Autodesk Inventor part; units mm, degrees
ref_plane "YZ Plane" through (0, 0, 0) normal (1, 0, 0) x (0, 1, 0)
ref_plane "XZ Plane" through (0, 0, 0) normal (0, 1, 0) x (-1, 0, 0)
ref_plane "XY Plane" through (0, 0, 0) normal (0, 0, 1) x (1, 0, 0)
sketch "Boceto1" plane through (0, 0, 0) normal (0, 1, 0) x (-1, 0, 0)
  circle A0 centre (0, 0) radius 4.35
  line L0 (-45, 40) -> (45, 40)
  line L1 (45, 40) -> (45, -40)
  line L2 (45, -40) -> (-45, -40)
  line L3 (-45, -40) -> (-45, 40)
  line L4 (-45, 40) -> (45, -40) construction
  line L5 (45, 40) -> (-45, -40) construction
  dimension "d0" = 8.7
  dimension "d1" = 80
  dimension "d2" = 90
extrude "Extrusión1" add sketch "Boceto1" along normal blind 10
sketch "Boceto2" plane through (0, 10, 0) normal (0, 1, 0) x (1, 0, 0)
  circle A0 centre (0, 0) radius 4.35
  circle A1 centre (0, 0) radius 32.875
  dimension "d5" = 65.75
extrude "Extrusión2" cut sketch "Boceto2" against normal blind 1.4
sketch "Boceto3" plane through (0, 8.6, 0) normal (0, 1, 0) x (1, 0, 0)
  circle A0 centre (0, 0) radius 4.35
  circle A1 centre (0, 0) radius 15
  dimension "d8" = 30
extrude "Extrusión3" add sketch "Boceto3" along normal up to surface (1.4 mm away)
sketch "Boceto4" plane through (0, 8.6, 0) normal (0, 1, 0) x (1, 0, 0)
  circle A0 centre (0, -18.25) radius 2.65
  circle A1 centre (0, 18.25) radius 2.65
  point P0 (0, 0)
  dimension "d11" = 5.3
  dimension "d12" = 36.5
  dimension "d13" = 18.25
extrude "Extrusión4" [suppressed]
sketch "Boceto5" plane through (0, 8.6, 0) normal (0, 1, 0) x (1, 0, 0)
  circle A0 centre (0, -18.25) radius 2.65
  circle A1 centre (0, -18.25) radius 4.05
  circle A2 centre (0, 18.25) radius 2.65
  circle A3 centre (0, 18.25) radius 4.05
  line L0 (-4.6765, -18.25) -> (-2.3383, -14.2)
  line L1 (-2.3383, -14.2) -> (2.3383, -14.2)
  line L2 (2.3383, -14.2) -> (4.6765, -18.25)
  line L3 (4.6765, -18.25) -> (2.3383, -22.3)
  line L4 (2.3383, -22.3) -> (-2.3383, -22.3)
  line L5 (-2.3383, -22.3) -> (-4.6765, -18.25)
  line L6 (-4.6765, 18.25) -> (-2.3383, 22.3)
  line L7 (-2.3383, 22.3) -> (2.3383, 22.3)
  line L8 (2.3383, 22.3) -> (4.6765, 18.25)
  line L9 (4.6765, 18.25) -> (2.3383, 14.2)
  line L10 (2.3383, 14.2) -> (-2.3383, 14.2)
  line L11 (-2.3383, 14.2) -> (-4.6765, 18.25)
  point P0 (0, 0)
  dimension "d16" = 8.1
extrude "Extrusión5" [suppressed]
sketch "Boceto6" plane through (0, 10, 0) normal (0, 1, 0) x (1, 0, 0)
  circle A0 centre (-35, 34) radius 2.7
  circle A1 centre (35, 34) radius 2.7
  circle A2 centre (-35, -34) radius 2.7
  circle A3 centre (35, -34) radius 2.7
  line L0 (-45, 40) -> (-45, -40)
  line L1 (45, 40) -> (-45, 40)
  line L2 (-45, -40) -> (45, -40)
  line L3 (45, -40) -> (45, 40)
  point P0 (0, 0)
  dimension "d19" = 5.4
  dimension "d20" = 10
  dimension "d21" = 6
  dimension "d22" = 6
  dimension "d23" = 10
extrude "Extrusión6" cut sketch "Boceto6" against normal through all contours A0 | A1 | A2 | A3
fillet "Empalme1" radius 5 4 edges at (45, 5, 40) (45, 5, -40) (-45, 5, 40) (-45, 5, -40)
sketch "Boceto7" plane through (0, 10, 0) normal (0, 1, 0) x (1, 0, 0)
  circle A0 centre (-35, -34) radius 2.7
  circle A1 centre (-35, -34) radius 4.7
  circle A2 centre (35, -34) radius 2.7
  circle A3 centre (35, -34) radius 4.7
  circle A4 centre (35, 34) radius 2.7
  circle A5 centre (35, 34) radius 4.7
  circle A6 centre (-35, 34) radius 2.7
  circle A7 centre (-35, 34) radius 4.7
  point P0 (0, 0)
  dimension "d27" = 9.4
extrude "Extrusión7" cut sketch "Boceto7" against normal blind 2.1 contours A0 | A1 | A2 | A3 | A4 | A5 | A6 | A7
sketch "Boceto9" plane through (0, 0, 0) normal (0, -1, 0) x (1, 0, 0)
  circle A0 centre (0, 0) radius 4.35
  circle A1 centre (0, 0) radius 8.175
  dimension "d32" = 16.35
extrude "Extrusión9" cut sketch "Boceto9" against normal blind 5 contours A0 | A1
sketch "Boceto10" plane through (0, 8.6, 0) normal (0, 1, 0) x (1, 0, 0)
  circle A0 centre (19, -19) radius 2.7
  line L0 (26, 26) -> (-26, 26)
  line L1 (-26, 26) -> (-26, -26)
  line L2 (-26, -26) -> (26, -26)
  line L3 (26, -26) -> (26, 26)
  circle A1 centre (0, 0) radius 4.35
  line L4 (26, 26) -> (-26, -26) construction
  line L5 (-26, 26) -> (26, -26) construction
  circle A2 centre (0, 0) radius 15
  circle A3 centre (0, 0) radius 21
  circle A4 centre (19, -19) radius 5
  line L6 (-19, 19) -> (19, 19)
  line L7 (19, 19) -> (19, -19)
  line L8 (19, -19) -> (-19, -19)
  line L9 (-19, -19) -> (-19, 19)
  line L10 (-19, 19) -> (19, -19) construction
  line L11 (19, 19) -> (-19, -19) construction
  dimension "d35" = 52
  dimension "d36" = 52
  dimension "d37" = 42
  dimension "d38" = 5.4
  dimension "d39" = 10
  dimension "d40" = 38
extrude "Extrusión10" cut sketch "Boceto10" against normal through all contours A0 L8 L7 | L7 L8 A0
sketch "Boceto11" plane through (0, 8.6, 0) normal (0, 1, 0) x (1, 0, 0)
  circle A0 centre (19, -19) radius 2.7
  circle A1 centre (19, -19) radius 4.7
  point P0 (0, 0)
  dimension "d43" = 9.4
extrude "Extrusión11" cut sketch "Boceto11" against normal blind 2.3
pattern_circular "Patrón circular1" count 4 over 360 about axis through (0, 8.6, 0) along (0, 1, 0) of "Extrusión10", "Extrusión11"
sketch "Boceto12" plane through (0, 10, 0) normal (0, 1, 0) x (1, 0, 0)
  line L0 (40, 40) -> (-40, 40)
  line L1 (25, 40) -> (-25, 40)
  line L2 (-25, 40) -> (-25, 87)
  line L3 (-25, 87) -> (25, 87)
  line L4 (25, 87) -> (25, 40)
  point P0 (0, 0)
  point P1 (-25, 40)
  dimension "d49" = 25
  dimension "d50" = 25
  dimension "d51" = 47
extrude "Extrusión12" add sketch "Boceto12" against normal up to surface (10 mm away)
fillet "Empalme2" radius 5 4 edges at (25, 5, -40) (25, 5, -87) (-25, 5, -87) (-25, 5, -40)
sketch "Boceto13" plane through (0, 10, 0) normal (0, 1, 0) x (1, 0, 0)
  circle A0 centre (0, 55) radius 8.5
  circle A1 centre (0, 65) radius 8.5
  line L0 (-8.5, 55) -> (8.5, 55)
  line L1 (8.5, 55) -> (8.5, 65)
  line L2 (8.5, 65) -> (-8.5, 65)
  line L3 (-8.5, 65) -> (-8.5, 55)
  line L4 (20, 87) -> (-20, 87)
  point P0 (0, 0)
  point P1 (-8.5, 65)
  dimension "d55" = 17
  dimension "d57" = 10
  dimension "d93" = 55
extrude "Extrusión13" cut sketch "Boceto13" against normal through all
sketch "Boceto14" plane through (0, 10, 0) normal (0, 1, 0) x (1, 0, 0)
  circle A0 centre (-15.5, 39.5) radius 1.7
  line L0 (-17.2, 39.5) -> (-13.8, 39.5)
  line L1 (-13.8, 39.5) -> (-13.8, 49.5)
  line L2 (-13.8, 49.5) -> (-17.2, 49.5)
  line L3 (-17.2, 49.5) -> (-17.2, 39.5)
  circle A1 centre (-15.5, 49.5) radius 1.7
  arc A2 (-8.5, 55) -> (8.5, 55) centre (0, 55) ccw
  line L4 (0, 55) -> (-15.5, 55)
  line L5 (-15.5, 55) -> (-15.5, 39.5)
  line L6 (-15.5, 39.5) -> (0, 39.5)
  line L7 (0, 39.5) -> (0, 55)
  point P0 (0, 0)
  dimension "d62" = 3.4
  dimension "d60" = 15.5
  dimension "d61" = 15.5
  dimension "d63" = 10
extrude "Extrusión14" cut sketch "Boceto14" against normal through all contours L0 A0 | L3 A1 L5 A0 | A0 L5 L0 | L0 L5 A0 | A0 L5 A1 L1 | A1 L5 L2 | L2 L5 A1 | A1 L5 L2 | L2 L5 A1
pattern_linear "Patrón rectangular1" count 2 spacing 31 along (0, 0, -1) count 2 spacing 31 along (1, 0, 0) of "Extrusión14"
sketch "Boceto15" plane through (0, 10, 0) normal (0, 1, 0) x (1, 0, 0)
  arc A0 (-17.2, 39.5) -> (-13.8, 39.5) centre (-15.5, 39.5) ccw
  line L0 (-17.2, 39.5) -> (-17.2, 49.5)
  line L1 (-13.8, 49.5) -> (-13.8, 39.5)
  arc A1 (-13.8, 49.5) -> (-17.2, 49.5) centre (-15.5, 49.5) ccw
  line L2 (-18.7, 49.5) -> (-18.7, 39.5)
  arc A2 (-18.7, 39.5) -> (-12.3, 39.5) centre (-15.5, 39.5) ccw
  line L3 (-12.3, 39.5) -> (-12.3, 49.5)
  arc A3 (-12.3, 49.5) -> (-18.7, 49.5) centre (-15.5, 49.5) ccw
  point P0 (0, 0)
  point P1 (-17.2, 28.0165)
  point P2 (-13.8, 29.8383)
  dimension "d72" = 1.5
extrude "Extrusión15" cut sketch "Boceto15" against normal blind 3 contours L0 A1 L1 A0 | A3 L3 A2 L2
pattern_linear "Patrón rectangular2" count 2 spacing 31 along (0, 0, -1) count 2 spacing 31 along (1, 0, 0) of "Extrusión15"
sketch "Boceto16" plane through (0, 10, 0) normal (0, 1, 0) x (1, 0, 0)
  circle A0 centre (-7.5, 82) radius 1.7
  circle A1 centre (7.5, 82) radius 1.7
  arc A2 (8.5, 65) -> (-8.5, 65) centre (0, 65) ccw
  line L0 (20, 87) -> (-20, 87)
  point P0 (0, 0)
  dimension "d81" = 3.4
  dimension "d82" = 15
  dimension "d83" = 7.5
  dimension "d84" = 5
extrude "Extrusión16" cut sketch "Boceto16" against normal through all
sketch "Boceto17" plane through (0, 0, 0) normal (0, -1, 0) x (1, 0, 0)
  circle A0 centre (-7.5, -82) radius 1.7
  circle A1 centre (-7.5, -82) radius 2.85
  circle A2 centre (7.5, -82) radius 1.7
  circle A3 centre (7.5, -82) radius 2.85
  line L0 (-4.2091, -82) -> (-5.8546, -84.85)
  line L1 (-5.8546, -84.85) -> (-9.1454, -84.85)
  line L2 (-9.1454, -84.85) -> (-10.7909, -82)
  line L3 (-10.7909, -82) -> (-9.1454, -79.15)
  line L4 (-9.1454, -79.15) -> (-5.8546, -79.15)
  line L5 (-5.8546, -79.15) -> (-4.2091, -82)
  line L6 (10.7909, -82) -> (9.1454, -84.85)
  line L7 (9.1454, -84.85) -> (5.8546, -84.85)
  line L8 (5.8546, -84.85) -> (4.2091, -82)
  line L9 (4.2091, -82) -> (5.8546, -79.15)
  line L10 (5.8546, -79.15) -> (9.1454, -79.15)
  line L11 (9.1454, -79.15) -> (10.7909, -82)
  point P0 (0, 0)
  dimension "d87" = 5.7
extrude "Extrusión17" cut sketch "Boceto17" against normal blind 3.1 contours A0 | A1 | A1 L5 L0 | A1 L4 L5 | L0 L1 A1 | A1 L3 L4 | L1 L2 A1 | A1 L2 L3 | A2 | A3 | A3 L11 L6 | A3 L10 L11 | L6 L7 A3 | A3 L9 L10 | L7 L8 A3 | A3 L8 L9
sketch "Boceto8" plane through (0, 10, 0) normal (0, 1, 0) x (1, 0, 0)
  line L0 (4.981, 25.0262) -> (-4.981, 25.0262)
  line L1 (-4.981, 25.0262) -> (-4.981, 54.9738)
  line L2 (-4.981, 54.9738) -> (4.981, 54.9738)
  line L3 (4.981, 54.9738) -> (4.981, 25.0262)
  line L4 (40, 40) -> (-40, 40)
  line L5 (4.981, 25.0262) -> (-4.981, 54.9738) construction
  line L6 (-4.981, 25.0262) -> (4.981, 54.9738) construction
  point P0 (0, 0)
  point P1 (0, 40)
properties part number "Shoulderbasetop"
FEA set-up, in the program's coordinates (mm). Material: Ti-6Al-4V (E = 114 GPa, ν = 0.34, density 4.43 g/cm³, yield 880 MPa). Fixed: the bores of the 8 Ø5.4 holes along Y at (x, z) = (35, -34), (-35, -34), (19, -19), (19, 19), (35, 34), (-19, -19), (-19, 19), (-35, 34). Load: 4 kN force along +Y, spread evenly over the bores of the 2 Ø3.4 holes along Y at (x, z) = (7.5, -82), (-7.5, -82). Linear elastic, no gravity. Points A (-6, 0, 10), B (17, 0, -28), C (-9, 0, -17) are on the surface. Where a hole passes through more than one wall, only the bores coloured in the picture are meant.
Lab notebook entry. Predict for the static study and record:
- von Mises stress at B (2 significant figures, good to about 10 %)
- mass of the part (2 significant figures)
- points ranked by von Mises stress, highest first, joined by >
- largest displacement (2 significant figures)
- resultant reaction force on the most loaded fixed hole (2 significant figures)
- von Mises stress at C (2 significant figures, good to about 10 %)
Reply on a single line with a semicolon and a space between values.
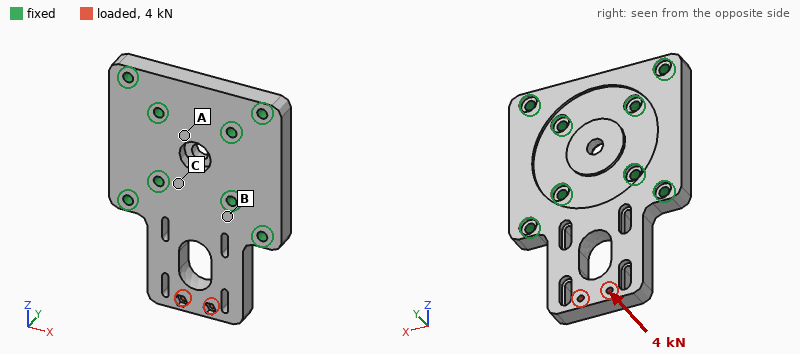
170 MPa; 360 g; B > C > A; 0.86 mm; 3.5 kN; 76 MPa
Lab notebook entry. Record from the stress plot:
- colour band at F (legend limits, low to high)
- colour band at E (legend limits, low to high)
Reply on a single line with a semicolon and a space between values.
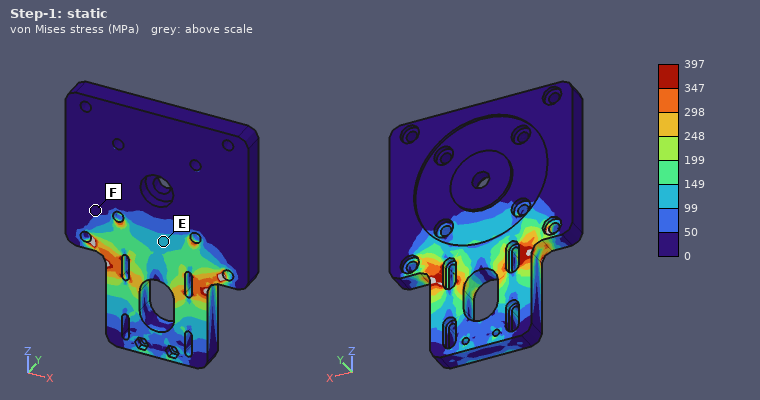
0 to 50 MPa; 99 to 149 MPa
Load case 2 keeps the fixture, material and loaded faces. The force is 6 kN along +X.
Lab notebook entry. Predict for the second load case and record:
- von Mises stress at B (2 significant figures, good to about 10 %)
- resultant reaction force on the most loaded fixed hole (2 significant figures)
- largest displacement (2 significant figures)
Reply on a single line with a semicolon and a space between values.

29 MPa; 3.5 kN; 84 µm
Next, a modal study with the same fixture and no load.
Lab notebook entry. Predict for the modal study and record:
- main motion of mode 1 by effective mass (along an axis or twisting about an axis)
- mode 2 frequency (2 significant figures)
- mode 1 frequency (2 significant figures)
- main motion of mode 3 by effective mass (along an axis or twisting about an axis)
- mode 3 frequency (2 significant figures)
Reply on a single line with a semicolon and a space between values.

along Y; 5100 Hz; 2100 Hz; along X; 7800 Hz
